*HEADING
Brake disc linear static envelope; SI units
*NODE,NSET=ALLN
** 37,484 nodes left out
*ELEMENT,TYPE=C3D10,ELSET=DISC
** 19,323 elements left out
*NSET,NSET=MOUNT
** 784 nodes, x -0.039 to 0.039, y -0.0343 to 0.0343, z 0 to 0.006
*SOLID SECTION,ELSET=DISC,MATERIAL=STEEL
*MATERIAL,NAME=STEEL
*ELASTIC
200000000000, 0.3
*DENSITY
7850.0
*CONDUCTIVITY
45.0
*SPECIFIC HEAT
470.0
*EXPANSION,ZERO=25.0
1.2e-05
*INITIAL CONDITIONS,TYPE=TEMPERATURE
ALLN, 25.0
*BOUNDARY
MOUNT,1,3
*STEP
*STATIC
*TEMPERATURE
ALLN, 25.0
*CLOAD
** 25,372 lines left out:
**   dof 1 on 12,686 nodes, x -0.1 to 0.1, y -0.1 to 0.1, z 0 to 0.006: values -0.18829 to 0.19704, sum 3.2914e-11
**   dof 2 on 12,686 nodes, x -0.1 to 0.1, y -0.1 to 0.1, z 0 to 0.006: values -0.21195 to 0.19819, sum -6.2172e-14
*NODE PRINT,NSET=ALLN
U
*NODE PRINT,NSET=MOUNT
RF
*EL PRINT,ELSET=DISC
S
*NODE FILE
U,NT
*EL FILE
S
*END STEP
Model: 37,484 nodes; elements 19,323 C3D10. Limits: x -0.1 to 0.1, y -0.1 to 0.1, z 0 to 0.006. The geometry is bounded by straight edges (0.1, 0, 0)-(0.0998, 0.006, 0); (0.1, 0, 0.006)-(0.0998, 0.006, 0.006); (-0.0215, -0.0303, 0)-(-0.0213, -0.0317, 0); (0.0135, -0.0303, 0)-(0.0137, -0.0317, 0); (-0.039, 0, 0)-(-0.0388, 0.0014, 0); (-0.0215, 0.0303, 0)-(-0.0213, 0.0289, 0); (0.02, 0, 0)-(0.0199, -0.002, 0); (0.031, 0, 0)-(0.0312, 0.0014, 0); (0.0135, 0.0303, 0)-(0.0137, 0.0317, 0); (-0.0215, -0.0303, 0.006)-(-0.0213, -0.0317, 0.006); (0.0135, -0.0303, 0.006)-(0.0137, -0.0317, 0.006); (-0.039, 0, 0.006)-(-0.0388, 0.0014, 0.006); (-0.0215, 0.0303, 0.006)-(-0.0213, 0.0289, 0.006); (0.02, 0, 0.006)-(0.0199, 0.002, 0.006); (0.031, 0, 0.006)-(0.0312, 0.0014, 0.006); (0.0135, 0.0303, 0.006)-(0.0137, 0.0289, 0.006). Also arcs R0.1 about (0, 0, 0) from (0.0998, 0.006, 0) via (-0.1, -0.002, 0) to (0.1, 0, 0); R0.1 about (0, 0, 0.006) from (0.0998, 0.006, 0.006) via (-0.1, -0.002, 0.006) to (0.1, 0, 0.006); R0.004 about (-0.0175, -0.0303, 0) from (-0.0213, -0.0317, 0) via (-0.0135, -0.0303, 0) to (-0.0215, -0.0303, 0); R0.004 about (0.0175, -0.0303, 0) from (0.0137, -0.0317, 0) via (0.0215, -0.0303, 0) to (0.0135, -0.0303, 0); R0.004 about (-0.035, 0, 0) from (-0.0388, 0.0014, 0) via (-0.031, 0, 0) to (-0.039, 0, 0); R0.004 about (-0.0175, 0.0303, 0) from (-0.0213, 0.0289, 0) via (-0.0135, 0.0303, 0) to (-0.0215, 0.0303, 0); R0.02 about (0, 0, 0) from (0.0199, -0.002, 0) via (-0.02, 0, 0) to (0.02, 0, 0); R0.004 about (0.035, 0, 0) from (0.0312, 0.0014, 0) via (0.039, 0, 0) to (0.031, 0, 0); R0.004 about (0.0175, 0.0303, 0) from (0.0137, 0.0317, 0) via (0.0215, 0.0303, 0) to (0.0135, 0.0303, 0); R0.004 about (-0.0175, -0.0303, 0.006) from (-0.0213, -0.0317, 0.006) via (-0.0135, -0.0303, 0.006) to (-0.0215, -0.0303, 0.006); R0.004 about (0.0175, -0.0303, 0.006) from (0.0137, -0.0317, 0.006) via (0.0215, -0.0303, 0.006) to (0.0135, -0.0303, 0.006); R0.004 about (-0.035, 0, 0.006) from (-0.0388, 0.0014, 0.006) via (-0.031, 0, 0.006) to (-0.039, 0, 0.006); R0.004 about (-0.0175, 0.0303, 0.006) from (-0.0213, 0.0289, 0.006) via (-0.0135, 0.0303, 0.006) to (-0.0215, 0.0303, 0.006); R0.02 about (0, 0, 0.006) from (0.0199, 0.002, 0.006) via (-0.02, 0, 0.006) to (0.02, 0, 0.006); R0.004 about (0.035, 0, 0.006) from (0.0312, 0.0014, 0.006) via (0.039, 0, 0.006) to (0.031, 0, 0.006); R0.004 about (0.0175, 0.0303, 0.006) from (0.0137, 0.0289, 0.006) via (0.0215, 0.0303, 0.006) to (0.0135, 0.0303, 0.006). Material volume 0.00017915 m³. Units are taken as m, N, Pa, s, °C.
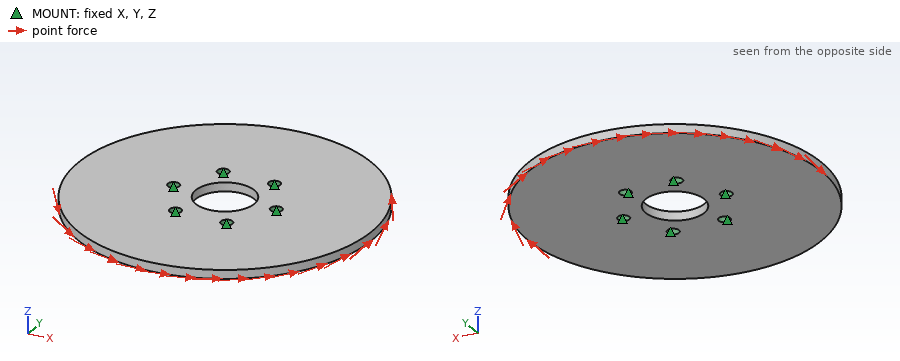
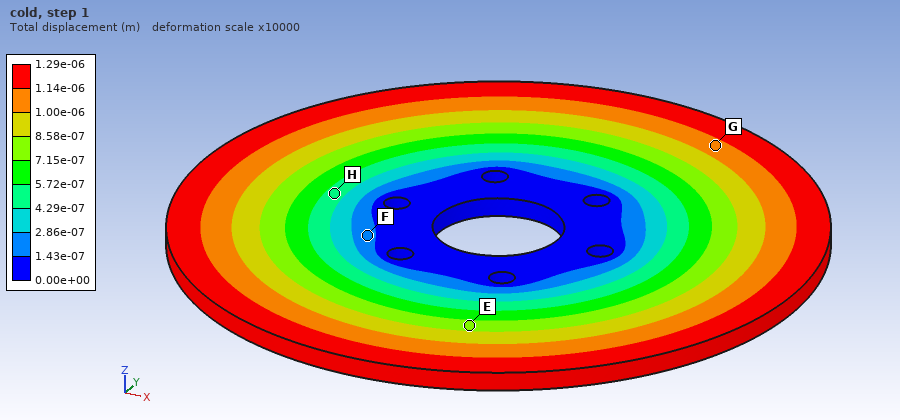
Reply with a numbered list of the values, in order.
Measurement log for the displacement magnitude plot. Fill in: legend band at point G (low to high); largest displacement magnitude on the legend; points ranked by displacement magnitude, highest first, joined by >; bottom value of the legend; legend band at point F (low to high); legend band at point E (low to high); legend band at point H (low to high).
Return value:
1. 1.00e-06 to 1.14e-06 m
2. 1.29e-06 m
3. G > E > H > F
4. 0.00e+00 m
5. 1.43e-07 to 2.86e-07 m
6. 7.15e-07 to 8.58e-07 m
7. 4.29e-07 to 5.72e-07 m
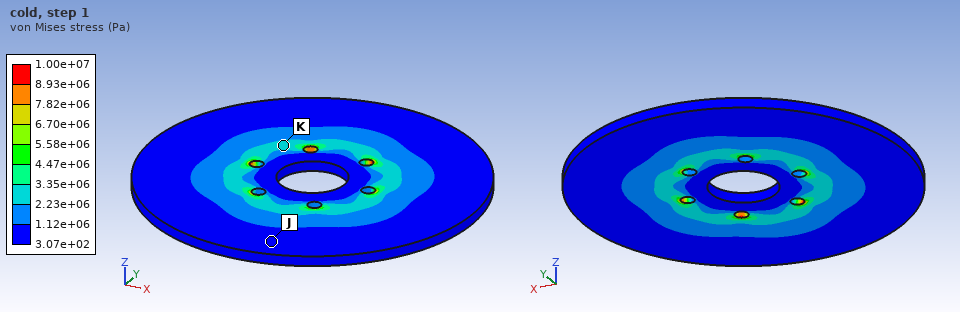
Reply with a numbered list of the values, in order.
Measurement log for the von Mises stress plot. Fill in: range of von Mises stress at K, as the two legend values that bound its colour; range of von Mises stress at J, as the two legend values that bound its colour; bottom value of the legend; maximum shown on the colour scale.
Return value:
1. 2.23e+06 to 3.35e+06 Pa
2. 3.07e+02 to 1.12e+06 Pa
3. 3.07e+02 Pa
4. 1.00e+07 Pa
